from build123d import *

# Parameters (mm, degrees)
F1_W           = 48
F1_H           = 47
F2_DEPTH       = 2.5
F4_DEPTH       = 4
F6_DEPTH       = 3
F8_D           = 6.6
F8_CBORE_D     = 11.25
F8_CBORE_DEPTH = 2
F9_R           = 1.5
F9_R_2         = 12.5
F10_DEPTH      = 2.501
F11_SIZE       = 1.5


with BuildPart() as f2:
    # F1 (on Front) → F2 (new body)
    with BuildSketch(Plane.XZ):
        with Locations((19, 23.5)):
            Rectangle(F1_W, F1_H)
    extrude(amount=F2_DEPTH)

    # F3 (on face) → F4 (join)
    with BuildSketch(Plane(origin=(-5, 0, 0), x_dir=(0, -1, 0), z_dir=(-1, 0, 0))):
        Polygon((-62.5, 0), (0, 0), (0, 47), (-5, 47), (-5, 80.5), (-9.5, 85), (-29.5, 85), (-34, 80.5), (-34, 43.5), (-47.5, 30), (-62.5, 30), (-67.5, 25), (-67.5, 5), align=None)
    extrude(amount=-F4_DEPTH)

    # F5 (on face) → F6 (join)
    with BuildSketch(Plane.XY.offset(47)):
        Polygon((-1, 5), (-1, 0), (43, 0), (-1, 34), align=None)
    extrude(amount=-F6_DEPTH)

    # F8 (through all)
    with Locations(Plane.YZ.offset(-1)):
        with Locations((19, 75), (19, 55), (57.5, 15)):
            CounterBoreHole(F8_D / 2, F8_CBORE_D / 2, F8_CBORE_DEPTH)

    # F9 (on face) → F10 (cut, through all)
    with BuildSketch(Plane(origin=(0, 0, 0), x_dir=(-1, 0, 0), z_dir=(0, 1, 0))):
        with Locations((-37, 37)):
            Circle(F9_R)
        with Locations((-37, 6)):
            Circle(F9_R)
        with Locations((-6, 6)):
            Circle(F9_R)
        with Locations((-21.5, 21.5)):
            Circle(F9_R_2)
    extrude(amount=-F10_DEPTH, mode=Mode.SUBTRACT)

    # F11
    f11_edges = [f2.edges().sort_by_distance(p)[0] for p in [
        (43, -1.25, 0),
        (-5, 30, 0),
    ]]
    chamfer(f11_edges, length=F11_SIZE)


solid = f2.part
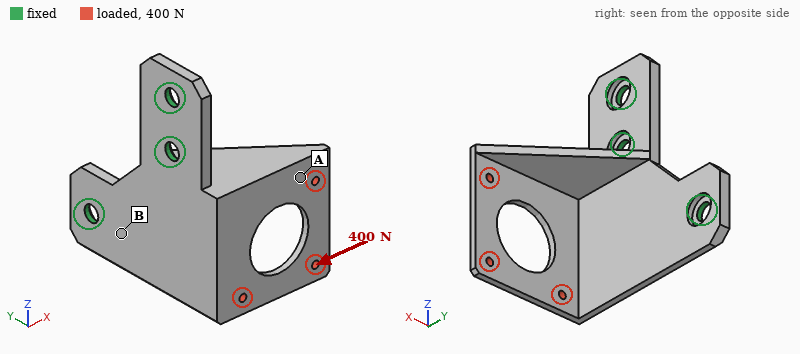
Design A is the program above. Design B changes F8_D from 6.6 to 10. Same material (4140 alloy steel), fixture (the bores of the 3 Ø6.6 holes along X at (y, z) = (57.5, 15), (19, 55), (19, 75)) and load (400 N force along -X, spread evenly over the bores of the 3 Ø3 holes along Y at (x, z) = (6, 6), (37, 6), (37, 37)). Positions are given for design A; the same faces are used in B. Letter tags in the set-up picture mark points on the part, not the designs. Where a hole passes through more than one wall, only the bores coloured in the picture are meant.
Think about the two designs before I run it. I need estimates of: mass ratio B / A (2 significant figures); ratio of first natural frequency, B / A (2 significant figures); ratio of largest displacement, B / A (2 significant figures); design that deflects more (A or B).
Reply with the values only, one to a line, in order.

0.99
1.1
0.78
A
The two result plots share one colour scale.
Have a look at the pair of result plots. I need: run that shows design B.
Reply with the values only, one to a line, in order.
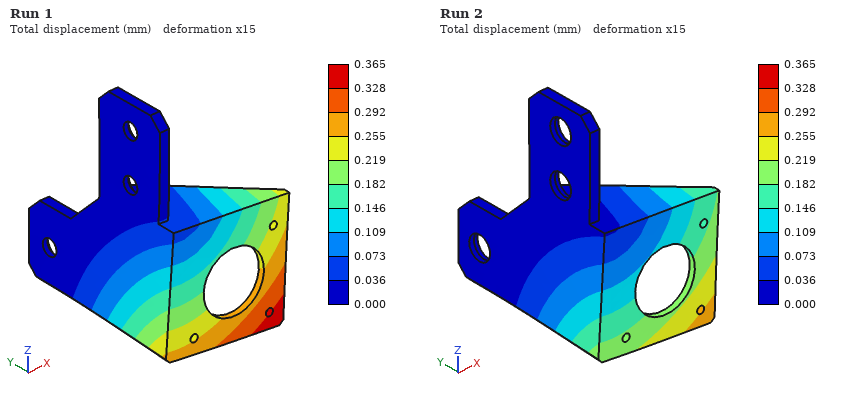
Run 2
